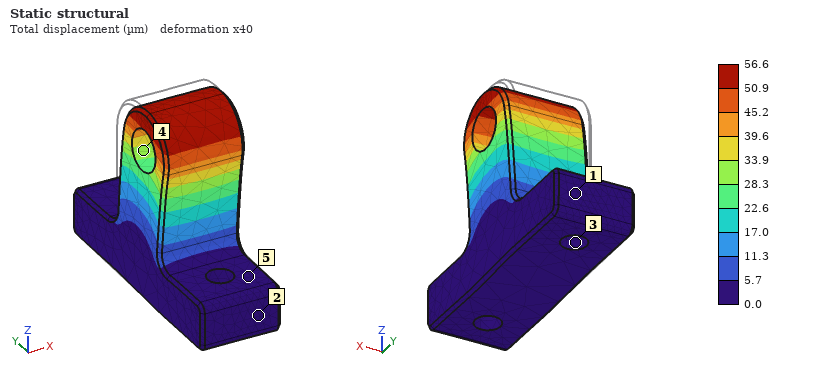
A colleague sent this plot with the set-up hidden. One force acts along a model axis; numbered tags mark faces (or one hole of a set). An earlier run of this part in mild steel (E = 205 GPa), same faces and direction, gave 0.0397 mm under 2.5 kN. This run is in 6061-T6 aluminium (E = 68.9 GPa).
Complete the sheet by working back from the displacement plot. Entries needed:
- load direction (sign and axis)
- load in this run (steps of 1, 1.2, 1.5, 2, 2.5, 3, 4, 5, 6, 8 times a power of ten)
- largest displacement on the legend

-Y
1.2 kN
56.6 µm
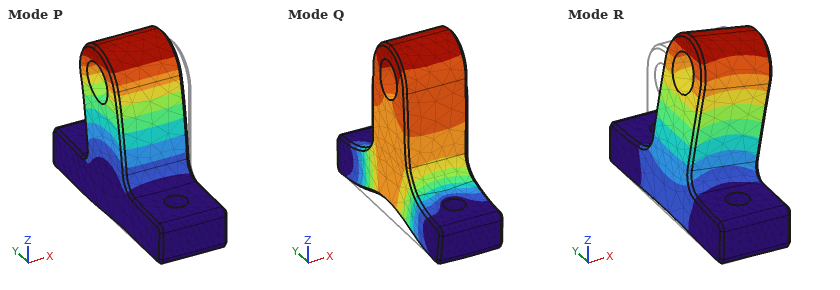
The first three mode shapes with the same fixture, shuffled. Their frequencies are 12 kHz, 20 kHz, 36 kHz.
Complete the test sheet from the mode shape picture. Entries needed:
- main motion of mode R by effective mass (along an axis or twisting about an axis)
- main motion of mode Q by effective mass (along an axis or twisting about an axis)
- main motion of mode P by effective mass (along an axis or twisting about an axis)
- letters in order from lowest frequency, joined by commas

along X
along Z
along Y
R, P, Q
